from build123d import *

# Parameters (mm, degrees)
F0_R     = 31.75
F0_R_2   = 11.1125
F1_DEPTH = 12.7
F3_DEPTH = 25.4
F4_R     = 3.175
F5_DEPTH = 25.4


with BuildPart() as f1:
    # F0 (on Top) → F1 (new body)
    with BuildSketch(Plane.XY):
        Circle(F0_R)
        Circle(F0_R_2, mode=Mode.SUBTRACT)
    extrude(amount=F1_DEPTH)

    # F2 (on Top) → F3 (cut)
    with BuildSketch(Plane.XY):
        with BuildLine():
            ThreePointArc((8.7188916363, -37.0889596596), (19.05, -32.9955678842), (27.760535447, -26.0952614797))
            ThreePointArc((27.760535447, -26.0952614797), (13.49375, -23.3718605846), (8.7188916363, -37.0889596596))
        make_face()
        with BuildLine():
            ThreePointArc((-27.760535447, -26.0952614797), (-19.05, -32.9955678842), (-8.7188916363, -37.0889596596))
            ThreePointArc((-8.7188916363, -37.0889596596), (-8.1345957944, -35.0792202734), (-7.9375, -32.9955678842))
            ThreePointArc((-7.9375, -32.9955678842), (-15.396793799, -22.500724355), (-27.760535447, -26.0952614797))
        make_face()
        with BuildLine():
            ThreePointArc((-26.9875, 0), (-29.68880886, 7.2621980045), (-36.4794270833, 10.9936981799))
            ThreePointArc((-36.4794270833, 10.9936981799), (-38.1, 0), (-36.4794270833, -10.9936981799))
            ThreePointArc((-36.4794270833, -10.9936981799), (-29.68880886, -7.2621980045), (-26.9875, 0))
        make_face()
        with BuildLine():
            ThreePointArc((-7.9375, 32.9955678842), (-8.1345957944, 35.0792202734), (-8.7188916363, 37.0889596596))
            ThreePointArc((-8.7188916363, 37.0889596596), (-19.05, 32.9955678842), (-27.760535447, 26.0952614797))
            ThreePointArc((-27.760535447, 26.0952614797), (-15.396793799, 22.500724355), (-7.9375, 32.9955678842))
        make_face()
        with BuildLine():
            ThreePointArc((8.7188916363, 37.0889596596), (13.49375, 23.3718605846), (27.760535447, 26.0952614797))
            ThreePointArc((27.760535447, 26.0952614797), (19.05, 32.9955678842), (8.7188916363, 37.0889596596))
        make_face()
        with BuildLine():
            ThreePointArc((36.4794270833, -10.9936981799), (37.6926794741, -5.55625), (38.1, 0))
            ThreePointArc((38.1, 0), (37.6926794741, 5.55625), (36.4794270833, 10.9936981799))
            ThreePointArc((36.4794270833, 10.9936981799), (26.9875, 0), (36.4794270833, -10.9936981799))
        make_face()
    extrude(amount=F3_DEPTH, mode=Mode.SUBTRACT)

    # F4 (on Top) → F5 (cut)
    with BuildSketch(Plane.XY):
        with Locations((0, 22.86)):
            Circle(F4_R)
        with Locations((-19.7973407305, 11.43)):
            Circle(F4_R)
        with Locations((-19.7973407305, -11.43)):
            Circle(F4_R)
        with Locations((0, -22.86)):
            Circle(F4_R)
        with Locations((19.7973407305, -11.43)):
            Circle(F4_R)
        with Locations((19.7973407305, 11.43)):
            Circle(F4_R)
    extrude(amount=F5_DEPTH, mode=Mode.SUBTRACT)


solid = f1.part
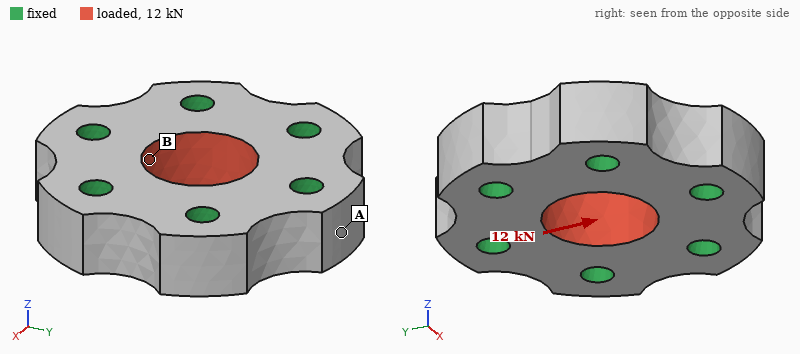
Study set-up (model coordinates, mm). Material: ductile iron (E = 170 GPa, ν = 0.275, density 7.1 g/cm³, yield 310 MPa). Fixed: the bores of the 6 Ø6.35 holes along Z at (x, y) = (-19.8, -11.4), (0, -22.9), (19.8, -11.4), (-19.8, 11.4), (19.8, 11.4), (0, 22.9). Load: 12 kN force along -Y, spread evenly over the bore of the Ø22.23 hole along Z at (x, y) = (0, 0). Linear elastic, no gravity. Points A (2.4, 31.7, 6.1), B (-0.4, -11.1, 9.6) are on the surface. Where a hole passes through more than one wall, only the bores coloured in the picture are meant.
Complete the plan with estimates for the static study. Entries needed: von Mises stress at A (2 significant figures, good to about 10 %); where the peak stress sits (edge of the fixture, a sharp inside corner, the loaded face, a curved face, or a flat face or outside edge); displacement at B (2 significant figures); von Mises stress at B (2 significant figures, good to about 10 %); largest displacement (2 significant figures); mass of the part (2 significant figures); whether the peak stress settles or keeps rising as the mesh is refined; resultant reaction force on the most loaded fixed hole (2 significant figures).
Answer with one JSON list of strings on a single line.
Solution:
["4.0 MPa", "edge of the fixture", "0.91 µm", "14 MPa", "1.2 µm", "200 g", "keeps rising", "2.9 kN"]
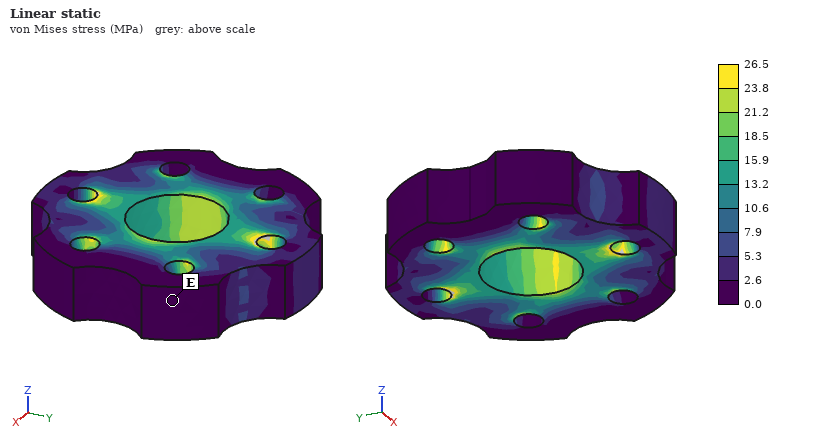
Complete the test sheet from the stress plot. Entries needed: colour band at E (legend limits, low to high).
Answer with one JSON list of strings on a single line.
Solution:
["0.0 to 2.6 MPa"]
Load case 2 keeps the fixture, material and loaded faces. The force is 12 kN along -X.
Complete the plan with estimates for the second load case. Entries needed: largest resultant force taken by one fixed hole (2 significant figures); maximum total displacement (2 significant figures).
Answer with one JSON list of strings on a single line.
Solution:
["2.6 kN", "1.2 µm"]
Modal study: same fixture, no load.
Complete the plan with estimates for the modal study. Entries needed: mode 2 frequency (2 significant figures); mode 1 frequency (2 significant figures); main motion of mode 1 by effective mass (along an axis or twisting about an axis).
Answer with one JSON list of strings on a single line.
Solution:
["59 kHz", "53 kHz", "along Z"]
